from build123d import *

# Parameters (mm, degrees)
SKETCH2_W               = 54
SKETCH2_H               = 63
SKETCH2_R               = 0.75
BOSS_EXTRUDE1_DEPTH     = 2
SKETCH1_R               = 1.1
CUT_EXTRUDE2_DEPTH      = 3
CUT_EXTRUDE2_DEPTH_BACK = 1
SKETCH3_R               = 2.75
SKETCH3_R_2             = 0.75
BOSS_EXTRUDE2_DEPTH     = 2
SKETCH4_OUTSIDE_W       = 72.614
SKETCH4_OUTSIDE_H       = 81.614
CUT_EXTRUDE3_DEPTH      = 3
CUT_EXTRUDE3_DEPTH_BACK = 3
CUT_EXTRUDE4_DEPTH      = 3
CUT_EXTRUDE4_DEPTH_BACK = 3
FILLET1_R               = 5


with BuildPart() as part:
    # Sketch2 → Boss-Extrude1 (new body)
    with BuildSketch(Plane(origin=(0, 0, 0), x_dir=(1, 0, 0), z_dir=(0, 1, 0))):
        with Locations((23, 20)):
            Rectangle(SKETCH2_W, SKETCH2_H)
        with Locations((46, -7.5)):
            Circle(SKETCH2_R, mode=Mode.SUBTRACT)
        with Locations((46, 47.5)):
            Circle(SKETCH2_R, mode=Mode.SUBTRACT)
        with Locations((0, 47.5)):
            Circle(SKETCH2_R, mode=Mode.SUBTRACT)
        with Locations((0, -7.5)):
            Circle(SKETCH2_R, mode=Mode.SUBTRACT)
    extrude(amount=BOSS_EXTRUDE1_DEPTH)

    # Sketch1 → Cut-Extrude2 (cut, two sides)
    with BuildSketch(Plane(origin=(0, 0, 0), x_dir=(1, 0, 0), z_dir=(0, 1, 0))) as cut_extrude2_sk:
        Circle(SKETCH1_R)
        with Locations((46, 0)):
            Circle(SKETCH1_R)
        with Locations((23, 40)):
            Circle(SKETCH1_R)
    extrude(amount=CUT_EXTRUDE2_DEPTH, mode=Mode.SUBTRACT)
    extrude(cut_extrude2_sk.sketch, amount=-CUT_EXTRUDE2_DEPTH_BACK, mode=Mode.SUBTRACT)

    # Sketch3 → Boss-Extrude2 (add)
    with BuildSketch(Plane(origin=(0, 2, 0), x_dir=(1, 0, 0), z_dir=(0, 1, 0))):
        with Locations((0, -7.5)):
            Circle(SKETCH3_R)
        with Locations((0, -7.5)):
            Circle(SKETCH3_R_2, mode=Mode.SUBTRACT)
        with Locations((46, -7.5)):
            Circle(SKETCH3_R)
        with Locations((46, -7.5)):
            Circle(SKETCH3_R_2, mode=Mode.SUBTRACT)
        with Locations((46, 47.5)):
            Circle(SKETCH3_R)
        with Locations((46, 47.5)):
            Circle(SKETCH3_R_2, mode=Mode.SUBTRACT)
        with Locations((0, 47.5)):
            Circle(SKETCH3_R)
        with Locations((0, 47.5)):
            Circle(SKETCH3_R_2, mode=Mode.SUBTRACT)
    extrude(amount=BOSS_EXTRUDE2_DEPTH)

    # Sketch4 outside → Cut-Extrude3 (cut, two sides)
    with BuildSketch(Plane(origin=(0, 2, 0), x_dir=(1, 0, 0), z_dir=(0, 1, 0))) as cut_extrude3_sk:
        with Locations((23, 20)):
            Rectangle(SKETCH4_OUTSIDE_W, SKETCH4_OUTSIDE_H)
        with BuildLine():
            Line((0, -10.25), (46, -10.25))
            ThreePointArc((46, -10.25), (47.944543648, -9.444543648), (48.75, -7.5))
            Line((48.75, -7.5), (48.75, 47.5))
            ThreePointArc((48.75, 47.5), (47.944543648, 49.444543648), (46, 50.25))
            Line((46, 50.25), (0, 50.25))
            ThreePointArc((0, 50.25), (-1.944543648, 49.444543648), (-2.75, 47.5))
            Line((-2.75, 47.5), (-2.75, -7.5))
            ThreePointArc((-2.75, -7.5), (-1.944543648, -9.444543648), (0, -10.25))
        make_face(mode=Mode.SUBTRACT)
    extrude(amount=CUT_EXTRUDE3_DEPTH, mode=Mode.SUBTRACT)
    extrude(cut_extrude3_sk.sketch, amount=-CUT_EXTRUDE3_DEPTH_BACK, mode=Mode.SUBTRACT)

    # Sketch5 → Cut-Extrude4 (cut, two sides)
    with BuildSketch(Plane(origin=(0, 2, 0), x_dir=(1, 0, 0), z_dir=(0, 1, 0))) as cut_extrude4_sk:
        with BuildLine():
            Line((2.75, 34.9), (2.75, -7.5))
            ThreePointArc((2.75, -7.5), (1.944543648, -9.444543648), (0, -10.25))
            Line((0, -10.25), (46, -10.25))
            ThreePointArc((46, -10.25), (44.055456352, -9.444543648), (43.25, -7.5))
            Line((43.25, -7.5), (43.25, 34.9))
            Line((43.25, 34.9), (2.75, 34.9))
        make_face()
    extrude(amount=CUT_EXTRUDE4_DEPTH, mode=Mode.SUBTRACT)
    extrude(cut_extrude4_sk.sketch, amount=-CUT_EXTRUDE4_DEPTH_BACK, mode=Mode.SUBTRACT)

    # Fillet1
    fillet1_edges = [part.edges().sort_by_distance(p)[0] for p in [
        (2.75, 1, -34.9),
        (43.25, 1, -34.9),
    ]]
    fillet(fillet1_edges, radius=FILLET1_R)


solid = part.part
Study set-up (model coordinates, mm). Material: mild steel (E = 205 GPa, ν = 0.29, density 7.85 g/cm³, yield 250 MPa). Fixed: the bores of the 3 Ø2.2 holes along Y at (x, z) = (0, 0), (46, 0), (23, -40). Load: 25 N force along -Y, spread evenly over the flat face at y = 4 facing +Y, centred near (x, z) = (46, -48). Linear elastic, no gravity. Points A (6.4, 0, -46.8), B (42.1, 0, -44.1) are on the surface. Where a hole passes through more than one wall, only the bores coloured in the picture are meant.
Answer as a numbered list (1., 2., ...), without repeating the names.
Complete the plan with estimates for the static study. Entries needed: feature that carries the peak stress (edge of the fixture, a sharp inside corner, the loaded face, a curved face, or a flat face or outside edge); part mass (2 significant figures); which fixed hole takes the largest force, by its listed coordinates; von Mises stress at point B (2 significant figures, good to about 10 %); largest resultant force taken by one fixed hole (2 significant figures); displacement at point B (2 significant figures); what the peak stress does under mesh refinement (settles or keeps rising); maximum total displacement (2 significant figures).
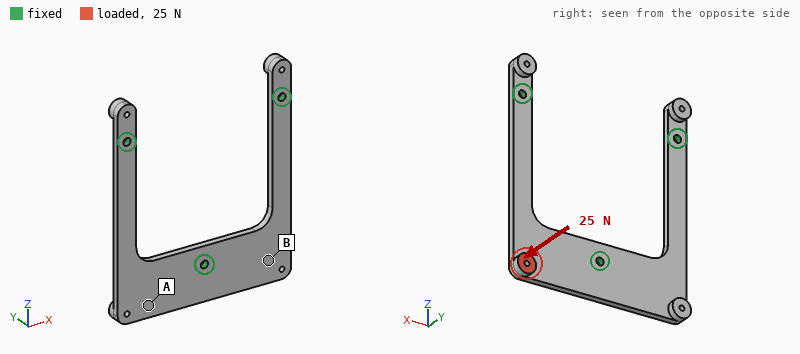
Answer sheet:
1. edge of the fixture
2. 21 g
3. (23, -40)
4. 13 MPa
5. 23 N
6. 34 µm
7. keeps rising
8. 58 µm
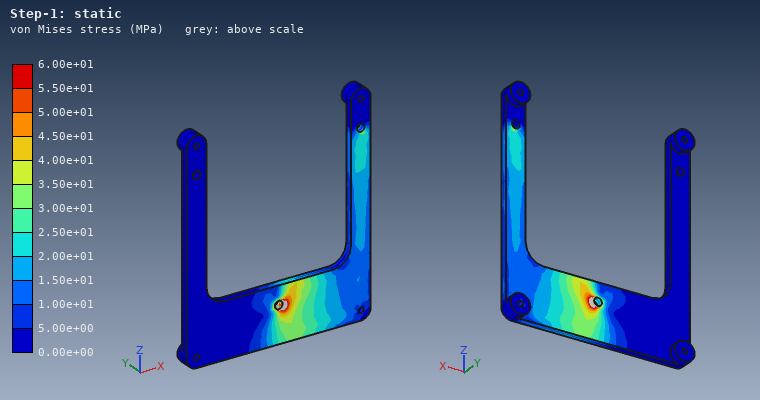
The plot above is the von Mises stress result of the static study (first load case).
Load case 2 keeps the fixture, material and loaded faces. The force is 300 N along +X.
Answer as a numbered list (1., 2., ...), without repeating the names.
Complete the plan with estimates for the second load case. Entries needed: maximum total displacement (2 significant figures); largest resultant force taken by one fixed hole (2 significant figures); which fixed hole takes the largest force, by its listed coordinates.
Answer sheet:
1. 0.12 mm
2. 310 N
3. (23, -40)
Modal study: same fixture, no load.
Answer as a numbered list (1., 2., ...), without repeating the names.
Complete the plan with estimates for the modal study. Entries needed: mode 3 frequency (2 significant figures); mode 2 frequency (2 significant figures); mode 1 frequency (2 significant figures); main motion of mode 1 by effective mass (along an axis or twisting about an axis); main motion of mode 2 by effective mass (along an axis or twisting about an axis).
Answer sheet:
1. 5100 Hz
2. 2400 Hz
3. 2100 Hz
4. twisting about Z
5. along Y
